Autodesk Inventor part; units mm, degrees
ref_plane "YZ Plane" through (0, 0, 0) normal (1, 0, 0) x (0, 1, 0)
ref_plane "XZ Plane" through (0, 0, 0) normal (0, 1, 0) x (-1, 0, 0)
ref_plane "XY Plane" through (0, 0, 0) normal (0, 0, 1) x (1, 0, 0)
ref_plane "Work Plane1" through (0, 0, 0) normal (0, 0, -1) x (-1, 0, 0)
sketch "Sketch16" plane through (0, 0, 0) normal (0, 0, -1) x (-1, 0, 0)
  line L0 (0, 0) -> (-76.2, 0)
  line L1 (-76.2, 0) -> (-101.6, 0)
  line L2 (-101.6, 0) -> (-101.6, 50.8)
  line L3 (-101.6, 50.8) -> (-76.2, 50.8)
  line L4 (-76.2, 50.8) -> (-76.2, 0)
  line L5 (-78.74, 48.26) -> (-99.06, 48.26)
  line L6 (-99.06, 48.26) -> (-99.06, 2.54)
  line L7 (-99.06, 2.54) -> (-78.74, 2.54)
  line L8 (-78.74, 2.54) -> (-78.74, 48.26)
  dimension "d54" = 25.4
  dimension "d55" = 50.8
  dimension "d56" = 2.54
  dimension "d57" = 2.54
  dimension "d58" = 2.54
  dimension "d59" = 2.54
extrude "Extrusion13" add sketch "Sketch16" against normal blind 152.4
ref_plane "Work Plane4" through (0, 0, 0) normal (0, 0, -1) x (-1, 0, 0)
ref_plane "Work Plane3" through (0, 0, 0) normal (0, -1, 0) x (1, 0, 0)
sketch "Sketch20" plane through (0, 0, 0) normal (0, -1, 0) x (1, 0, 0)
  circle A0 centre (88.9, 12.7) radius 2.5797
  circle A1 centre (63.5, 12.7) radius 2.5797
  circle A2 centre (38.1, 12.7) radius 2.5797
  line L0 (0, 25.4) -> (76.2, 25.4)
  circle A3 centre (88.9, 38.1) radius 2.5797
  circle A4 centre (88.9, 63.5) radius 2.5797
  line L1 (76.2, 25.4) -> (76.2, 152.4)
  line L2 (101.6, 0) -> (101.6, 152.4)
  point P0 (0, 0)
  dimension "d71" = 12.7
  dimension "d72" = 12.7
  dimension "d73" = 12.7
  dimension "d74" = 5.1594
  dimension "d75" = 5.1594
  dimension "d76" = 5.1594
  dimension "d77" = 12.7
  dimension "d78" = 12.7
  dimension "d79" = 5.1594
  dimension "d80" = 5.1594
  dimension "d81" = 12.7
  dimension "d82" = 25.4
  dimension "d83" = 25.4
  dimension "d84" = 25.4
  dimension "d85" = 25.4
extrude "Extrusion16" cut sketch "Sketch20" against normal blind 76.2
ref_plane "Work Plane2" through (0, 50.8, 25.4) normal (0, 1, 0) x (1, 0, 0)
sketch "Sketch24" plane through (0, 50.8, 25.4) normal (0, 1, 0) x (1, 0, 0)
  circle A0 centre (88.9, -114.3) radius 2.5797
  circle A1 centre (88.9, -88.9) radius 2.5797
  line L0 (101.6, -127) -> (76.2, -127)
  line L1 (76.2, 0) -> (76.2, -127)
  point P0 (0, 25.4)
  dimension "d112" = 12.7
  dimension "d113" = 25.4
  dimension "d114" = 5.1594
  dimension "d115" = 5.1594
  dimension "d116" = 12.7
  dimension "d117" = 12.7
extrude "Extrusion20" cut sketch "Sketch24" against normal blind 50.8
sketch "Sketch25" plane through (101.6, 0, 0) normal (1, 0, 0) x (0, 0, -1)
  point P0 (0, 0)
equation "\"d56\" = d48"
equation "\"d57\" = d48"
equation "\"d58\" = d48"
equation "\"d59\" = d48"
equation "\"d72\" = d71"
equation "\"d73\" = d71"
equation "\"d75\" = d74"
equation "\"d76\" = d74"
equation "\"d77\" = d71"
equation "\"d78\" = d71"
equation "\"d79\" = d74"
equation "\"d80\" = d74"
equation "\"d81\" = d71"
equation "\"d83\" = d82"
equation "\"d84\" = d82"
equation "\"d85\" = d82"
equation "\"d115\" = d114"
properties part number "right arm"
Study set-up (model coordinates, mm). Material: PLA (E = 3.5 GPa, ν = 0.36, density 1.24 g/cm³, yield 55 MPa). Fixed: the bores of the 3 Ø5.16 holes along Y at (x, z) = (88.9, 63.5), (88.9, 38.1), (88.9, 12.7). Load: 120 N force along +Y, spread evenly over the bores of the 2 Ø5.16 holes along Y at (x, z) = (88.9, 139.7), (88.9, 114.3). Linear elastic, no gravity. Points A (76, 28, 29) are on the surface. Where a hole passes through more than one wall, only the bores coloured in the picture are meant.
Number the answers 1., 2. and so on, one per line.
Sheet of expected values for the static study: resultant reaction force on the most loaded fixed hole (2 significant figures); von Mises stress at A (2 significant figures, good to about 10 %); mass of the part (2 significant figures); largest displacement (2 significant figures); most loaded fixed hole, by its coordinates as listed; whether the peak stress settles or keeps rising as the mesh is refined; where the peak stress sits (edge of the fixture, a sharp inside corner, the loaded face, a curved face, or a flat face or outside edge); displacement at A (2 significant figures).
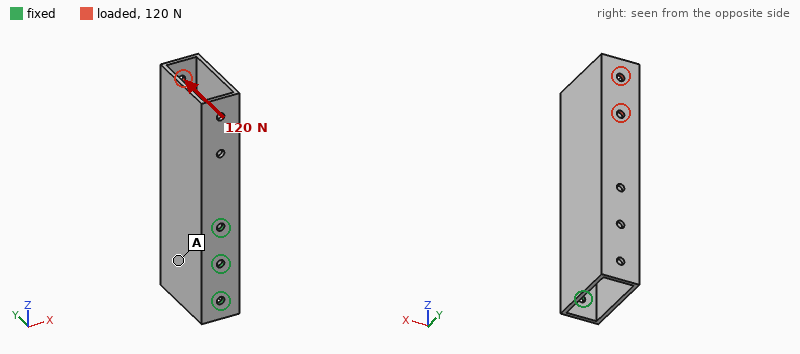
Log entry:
1. 250 N
2. 2.1 MPa
3. 68 g
4. 1.0 mm
5. (88.9, 63.5)
6. keeps rising
7. edge of the fixture
8. 0.18 mm
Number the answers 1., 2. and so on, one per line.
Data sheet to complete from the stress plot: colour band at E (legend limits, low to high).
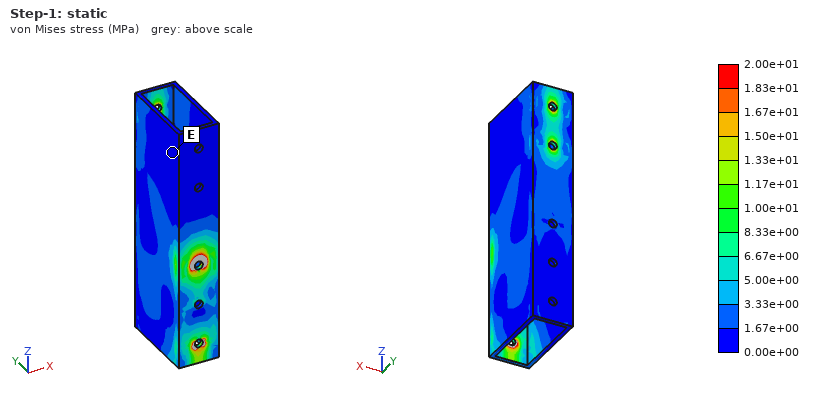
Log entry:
1. 0.00e+00 to 1.67e+00 MPa
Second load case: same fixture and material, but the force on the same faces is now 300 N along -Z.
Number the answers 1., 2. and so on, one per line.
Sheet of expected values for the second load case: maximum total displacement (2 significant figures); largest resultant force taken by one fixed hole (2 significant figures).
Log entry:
1. 1.3 mm
2. 280 N
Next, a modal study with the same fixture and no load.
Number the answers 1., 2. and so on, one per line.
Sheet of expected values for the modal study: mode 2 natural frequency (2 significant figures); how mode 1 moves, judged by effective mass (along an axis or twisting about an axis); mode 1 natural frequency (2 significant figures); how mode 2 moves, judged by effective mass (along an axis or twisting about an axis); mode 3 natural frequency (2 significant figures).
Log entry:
1. 350 Hz
2. along X
3. 190 Hz
4. along Y
5. 460 Hz
